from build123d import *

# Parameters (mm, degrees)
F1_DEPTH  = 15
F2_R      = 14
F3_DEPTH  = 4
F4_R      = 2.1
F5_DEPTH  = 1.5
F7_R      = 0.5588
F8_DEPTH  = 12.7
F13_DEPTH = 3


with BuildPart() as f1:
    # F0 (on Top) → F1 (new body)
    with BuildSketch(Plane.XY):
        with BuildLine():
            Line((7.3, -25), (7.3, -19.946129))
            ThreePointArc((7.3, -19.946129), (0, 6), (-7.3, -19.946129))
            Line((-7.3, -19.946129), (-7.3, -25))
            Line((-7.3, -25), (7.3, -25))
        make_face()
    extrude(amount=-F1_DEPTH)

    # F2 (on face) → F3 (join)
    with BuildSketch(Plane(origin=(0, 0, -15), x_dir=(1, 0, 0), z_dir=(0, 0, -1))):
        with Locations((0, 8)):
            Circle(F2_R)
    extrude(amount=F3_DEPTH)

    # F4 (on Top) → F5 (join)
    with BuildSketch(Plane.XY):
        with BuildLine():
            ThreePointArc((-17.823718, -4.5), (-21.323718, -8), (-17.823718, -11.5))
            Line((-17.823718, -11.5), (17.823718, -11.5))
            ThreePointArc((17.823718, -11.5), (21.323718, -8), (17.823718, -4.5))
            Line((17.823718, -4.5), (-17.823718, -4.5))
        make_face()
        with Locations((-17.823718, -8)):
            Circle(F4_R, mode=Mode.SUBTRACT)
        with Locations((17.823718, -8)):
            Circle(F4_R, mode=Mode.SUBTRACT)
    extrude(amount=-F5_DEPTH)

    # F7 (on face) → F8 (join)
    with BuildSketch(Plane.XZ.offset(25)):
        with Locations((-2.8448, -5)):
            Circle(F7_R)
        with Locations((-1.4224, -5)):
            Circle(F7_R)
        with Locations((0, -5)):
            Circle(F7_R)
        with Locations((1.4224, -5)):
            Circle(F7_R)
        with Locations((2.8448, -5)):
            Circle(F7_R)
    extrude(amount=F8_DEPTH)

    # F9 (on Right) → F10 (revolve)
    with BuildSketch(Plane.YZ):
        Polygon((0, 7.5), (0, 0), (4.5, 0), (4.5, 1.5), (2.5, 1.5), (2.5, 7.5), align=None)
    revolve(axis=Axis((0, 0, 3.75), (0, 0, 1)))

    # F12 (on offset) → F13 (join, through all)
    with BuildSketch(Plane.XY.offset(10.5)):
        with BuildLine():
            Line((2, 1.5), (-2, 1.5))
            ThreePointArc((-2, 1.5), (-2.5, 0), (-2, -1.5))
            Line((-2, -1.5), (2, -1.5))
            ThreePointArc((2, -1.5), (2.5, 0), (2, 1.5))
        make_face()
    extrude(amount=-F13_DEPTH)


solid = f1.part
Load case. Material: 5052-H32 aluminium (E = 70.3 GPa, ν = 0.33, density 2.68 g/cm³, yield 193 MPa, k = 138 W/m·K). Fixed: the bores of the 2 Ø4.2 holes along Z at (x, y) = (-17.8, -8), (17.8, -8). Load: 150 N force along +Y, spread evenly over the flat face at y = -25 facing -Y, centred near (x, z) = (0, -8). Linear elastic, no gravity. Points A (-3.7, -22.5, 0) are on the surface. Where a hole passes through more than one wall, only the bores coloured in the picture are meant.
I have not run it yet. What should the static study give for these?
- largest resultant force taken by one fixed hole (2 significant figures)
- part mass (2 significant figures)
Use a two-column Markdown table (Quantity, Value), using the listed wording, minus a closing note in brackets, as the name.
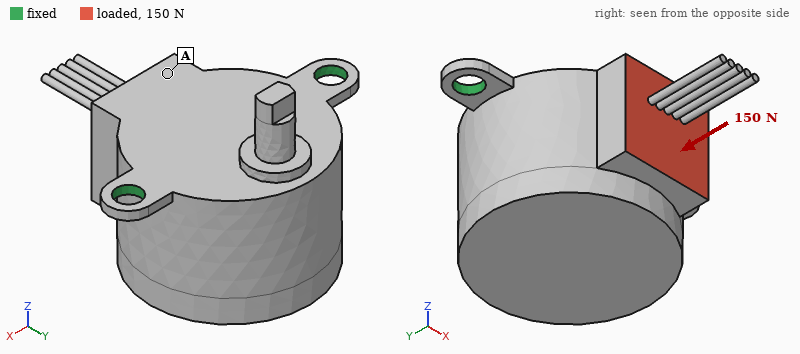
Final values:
| Quantity | Value |
|---|---|
| largest resultant force taken by one fixed hole | 75 N |
| part mass | 35 g |
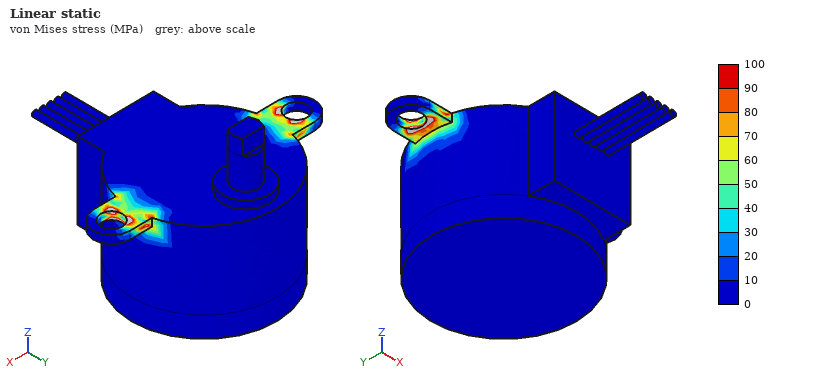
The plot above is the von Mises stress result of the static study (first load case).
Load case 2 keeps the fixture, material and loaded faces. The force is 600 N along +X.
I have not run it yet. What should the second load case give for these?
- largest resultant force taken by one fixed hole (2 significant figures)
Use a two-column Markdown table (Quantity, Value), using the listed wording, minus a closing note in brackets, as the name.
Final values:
| Quantity | Value |
|---|---|
| largest resultant force taken by one fixed hole | 460 N |
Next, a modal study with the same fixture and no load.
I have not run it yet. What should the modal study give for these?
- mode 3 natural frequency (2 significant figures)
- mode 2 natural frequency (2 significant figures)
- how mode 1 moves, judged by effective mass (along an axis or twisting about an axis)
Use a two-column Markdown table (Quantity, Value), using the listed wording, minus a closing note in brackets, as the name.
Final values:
| Quantity | Value |
|---|---|
| mode 3 natural frequency | 4800 Hz |
| mode 2 natural frequency | 4800 Hz |
| how mode 1 moves, judged by effective mass | along Y |
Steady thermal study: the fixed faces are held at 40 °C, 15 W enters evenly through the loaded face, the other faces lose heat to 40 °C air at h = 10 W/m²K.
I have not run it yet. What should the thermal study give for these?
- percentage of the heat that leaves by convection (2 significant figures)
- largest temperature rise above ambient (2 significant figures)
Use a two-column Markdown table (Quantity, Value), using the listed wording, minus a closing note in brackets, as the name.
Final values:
| Quantity | Value |
|---|---|
| percentage of the heat that leaves by convection | 4.8 % |
| largest temperature rise above ambient | 27 K |
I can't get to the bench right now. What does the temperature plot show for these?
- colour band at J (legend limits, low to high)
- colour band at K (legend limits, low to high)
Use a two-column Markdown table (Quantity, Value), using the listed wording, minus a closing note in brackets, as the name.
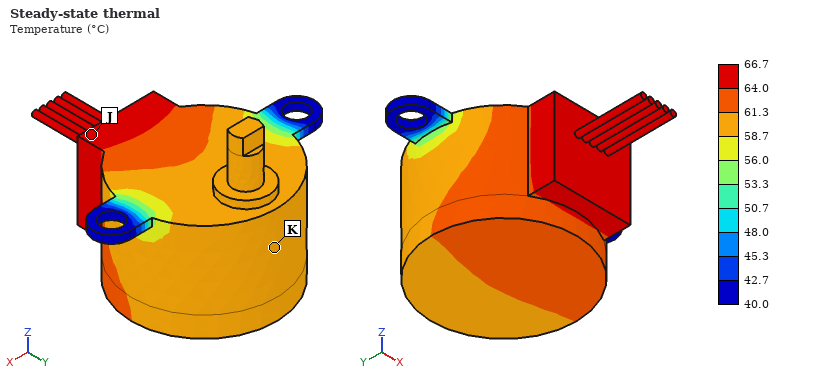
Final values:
| Quantity | Value |
|---|---|
| colour band at J | 64.0 to 66.7 °C |
| colour band at K | 58.7 to 61.3 °C |
